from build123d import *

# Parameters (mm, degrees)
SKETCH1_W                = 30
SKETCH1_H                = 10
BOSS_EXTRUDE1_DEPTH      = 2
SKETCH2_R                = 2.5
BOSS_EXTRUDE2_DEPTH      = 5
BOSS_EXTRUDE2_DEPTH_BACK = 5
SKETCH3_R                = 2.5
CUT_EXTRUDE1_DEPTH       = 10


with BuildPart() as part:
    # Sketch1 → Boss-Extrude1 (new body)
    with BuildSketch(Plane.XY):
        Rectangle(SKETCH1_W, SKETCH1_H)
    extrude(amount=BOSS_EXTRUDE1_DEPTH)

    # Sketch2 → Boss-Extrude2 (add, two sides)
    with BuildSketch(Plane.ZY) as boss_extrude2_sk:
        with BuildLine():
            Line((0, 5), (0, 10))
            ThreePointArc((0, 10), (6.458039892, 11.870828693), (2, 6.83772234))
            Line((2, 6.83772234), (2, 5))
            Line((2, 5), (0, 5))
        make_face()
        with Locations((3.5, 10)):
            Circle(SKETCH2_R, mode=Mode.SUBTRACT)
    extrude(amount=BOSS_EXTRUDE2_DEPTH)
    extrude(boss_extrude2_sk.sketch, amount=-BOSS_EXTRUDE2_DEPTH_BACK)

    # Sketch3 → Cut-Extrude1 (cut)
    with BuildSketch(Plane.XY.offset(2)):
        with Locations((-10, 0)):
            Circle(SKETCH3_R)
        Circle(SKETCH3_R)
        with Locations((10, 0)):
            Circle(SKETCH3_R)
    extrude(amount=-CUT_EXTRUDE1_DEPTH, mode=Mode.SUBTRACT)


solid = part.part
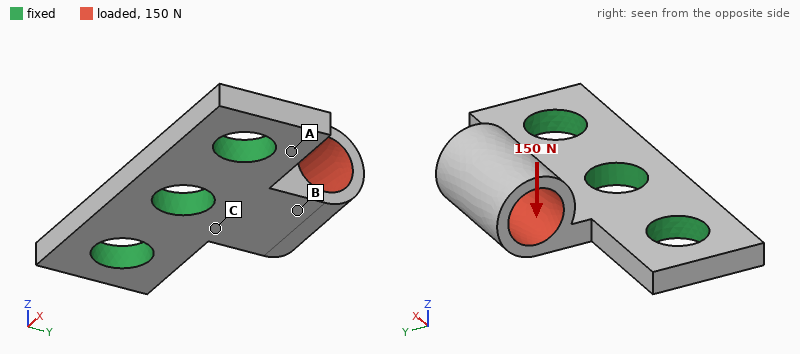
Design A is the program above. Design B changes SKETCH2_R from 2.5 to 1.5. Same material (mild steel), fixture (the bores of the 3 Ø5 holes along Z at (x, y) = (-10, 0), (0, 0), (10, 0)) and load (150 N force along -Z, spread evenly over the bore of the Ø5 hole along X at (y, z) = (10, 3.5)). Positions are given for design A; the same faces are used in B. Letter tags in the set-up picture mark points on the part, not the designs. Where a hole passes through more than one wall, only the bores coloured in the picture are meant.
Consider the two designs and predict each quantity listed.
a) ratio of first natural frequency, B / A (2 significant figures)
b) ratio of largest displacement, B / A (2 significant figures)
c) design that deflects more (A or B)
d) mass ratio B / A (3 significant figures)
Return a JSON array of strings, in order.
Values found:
["0.87", "0.86", "A", "1.17"]
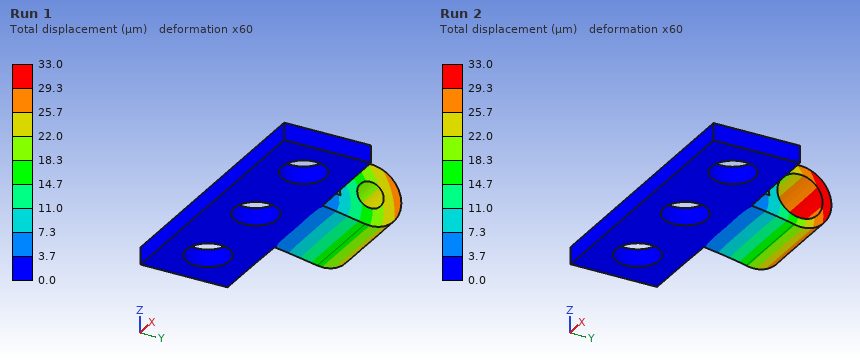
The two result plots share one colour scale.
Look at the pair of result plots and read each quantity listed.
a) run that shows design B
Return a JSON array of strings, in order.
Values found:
["Run 1"]
